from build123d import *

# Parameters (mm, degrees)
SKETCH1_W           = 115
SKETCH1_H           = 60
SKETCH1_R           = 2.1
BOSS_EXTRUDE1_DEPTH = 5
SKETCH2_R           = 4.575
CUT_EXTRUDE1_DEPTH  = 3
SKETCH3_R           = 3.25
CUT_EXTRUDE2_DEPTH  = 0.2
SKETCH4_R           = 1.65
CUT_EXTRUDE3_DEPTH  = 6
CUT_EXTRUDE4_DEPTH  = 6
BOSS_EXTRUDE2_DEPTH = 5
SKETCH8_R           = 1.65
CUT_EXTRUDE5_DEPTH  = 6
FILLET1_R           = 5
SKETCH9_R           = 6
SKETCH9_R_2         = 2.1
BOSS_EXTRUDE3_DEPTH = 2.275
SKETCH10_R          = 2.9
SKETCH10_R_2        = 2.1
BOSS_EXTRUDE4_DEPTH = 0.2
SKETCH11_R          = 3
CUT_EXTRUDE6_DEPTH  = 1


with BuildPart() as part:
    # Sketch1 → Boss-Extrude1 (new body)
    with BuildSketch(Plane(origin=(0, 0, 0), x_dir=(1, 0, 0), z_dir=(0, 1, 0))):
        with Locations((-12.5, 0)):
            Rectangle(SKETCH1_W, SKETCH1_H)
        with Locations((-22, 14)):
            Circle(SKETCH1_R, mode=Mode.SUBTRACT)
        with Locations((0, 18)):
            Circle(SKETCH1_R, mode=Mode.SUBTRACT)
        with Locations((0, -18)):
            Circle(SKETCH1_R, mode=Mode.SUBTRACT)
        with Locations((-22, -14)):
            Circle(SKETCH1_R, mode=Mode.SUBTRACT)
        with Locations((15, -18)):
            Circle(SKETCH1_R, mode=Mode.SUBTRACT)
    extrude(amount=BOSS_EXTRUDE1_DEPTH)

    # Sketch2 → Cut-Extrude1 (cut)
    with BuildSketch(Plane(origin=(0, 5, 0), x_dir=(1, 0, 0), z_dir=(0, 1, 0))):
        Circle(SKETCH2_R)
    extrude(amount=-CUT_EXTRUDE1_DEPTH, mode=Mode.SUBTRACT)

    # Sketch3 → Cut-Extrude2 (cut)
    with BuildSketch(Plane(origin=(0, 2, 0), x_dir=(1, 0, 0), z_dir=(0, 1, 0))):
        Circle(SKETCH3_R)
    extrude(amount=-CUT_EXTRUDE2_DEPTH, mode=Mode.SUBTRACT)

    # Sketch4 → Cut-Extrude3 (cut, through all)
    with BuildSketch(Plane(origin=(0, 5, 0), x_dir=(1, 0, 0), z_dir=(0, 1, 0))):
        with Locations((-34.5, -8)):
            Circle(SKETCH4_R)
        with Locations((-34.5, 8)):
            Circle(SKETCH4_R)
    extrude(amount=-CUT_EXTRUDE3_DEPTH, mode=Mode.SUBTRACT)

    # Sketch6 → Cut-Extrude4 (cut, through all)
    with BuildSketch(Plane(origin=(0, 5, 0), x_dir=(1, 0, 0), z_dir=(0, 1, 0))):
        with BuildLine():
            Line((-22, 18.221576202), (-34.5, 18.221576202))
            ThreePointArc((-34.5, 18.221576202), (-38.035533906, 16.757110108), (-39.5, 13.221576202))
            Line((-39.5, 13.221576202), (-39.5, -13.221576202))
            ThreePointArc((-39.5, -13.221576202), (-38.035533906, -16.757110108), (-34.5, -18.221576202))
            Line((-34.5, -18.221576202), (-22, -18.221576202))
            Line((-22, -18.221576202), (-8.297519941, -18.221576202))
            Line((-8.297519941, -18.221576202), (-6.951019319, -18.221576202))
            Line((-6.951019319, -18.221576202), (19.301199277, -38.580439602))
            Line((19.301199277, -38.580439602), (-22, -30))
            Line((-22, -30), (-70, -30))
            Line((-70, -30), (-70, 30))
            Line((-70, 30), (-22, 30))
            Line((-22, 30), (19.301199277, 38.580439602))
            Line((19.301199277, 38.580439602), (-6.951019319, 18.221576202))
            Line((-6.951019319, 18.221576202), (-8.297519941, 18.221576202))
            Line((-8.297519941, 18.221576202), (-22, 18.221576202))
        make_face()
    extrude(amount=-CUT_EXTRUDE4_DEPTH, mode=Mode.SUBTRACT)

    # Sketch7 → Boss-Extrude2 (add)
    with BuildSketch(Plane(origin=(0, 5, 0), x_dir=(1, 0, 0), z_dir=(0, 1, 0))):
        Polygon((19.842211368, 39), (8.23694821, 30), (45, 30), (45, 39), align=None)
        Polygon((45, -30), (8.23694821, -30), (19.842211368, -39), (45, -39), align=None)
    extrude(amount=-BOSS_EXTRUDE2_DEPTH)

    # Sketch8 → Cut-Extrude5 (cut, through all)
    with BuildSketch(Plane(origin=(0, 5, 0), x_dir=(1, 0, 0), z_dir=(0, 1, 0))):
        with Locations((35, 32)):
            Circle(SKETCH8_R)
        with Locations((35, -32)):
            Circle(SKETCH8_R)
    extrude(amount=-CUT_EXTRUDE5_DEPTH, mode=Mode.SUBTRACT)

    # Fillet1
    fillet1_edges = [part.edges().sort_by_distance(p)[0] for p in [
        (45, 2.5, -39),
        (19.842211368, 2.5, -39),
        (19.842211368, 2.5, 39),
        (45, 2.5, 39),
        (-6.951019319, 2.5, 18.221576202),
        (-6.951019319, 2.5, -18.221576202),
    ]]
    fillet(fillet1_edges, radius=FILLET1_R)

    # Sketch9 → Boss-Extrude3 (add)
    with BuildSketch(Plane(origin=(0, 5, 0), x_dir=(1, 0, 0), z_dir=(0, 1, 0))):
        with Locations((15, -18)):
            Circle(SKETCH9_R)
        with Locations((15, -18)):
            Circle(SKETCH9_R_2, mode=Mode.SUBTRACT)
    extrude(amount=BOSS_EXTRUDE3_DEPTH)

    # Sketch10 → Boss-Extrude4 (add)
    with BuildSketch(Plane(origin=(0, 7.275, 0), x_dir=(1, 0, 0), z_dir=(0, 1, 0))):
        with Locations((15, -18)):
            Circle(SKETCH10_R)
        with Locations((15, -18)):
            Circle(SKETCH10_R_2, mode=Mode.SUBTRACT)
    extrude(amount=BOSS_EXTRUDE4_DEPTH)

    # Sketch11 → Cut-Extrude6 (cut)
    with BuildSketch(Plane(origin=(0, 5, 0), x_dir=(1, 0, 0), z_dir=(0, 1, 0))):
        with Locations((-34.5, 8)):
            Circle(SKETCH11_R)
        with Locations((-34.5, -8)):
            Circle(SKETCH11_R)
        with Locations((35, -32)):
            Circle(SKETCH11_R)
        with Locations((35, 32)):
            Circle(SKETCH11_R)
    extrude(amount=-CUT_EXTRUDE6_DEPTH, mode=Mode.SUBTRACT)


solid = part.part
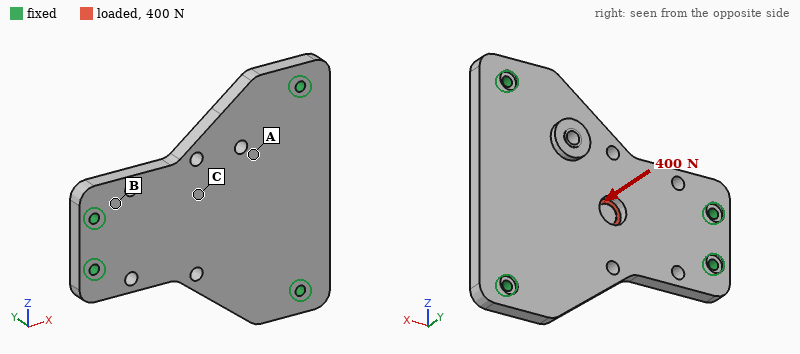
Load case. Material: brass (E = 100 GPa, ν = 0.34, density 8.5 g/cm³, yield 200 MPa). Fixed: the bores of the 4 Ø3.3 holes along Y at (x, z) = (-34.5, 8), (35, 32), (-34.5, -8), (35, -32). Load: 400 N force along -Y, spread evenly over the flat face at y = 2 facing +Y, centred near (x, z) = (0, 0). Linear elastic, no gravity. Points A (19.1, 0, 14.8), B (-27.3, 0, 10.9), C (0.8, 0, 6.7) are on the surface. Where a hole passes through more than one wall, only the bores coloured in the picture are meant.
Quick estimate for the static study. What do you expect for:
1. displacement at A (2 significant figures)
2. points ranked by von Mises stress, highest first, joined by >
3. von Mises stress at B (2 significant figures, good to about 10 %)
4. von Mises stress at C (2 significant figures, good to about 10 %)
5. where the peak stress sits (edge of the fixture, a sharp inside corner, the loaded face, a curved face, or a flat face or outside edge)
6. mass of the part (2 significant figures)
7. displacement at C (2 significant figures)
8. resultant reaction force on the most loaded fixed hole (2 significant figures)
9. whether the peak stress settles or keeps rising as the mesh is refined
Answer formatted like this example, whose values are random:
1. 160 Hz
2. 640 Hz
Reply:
1. 15 µm
2. C > B > A
3. 12 MPa
4. 22 MPa
5. edge of the fixture
6. 190 g
7. 27 µm
8. 110 N
9. keeps rising
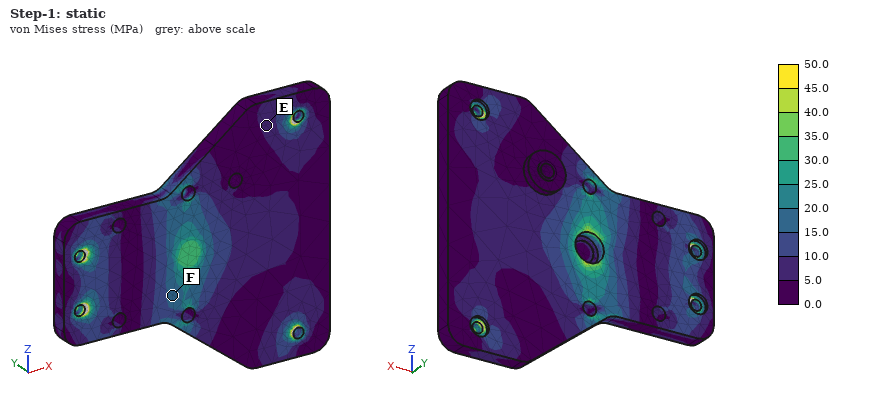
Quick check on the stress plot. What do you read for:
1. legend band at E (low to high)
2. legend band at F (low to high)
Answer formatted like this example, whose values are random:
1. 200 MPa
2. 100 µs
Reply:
1. 5.0 to 10.0 MPa
2. 15.0 to 20.0 MPa
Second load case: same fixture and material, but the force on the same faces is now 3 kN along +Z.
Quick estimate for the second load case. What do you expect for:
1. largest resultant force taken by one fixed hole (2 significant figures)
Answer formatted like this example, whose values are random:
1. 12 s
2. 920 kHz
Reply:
1. 1.3 kN
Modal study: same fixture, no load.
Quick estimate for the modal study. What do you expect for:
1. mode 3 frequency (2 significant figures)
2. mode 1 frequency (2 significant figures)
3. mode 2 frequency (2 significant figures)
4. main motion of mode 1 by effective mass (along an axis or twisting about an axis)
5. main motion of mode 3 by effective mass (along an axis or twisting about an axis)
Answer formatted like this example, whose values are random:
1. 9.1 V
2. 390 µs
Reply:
1. 4200 Hz
2. 2500 Hz
3. 4100 Hz
4. along Y
5. twisting about X
